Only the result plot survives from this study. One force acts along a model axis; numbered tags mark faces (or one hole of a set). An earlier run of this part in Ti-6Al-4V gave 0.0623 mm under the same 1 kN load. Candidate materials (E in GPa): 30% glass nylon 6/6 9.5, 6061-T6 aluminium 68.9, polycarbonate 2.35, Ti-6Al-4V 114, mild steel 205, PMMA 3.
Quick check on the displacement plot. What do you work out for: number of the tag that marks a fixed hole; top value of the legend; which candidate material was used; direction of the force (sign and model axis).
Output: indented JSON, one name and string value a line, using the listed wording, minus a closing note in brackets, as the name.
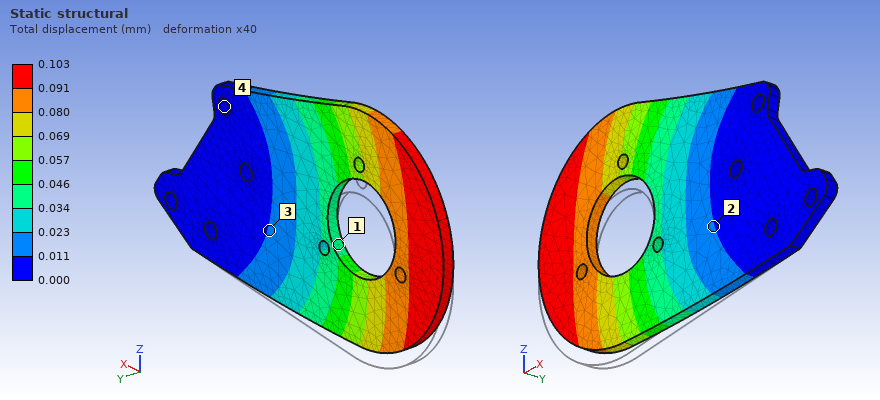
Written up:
{
  "number of the tag that marks a fixed hole": "4",
  "top value of the legend": "0.103 mm",
  "which candidate material was used": "6061-T6 aluminium",
  "direction of the force": "+Z"
}
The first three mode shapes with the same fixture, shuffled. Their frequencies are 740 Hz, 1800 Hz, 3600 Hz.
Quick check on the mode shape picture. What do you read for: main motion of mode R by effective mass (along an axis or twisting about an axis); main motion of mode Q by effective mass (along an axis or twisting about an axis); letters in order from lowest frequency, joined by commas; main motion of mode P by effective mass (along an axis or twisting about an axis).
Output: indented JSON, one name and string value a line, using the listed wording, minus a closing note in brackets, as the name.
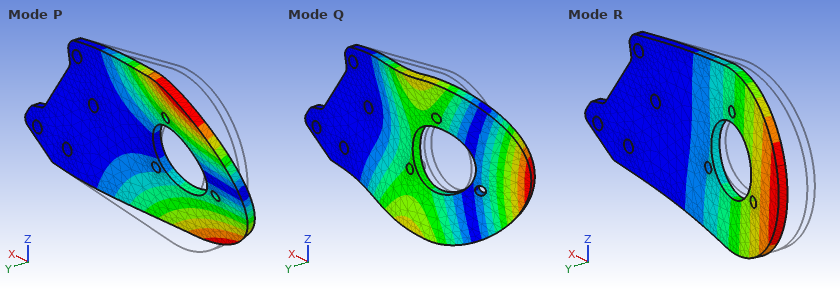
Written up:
{
  "main motion of mode R by effective mass": "along Y",
  "main motion of mode Q by effective mass": "along Y",
  "letters in order from lowest frequency, joined by commas": "R, P, Q",
  "main motion of mode P by effective mass": "twisting about X"
}
